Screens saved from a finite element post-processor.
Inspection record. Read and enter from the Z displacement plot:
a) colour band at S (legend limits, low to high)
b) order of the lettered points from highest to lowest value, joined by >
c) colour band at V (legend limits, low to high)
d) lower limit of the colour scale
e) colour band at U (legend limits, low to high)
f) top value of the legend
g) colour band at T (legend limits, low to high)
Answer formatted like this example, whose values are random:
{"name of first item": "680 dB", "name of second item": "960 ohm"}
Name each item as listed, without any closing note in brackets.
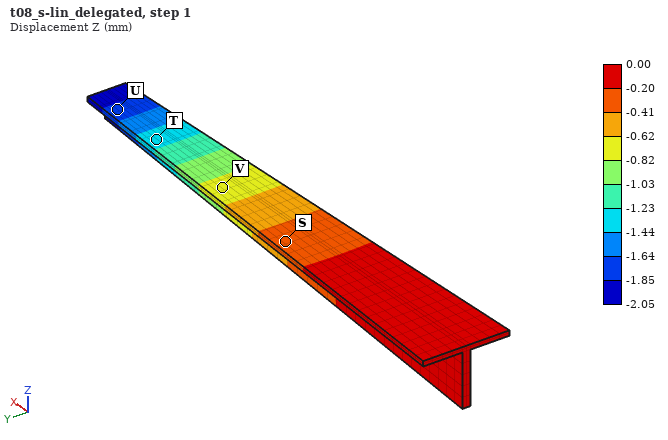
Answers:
{"colour band at S": "-0.41 to -0.20 mm", "order of the lettered points from highest to lowest value, joined by >": "S > V > T > U", "colour band at V": "-0.82 to -0.62 mm", "lower limit of the colour scale": "-2.05 mm", "colour band at U": "-1.85 to -1.64 mm", "top value of the legend": "0.00 mm", "colour band at T": "-1.44 to -1.23 mm"}
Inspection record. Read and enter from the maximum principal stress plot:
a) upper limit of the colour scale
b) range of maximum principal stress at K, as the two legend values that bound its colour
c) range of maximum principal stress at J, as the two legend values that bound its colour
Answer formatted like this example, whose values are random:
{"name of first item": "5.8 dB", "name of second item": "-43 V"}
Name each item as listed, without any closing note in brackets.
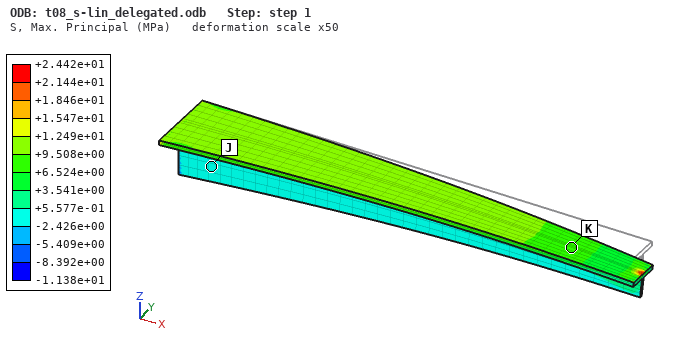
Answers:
{"upper limit of the colour scale": "+2.442e+01 MPa", "range of maximum principal stress at K, as the two legend values that bound its colour": "+6.524e+00 to +9.508e+00 MPa", "range of maximum principal stress at J, as the two legend values that bound its colour": "-2.426e+00 to +5.577e-01 MPa"}
